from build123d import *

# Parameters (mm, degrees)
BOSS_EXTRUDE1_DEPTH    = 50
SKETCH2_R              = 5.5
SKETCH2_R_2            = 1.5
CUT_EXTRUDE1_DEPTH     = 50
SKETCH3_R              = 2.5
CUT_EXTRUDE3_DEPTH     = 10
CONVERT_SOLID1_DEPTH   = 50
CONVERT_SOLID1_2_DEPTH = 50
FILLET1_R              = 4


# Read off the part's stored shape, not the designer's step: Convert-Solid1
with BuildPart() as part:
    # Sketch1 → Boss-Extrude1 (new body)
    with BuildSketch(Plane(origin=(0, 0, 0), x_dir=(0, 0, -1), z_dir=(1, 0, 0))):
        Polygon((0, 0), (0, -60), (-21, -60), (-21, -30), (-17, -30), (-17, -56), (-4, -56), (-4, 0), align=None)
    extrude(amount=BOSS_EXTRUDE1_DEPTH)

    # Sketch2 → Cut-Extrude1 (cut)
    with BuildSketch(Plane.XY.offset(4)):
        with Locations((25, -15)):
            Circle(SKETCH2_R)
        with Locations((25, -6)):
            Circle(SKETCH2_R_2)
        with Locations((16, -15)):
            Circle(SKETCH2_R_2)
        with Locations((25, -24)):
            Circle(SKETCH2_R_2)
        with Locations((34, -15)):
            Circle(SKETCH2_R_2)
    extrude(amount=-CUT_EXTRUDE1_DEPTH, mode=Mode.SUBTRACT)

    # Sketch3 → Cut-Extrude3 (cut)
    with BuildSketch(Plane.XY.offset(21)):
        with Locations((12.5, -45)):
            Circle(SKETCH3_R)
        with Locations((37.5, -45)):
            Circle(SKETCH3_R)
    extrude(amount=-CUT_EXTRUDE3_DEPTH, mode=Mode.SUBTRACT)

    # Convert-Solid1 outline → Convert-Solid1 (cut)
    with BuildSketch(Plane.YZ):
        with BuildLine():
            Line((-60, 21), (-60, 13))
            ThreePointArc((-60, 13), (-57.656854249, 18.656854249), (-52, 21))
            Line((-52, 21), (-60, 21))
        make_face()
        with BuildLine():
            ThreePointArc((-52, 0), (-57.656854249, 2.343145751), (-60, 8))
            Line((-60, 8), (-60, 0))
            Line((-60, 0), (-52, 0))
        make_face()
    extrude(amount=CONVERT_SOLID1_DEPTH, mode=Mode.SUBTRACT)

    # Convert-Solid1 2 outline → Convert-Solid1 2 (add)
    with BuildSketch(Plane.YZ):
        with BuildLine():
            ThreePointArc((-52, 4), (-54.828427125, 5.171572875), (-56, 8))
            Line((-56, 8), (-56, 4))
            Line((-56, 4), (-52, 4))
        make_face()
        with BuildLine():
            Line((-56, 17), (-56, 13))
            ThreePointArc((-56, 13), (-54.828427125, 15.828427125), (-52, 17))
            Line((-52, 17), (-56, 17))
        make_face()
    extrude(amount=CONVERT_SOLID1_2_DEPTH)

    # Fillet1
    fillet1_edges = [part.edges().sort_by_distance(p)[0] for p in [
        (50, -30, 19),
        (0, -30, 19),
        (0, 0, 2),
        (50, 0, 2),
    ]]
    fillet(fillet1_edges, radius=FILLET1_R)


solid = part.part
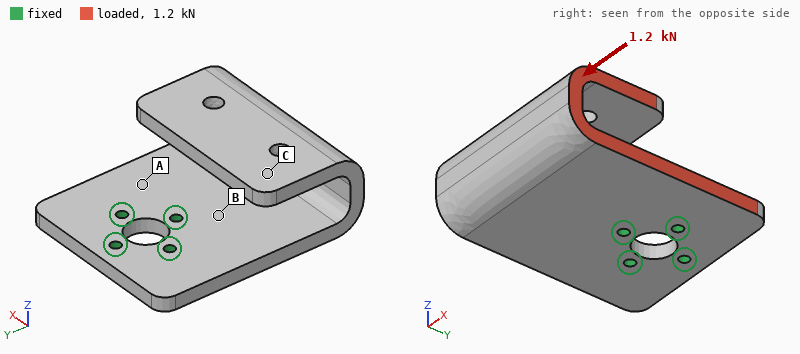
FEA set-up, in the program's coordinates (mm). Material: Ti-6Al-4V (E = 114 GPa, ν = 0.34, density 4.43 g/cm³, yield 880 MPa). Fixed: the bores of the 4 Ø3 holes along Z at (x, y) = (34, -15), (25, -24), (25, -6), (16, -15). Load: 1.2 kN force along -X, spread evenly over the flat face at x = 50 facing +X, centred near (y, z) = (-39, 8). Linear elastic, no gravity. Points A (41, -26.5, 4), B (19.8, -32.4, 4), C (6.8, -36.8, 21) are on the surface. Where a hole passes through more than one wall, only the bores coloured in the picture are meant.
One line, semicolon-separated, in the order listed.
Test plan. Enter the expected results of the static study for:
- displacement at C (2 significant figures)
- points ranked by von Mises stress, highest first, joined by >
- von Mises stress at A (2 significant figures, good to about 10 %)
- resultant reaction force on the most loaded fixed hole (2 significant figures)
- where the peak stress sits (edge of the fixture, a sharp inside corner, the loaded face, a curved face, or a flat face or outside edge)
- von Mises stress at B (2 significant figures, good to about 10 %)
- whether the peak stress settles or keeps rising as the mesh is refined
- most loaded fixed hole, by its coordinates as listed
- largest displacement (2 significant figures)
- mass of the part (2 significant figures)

0.15 mm; B > A > C; 30 MPa; 1.2 kN; edge of the fixture; 51 MPa; keeps rising; (25, -24); 0.17 mm; 84 g
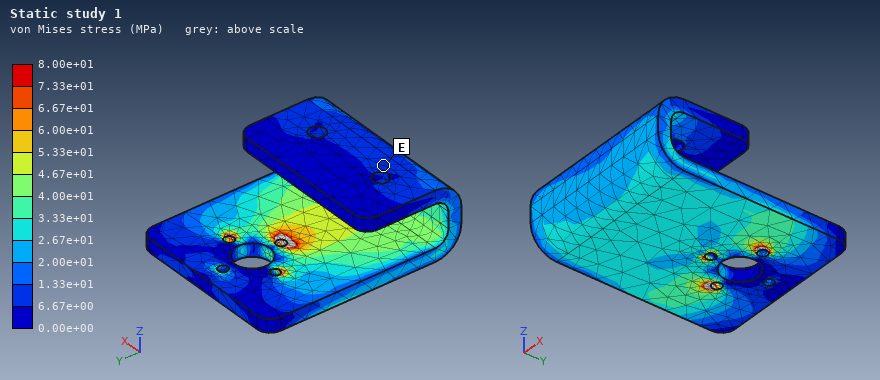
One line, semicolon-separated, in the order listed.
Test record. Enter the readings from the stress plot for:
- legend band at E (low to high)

6.67e+00 to 1.33e+01 MPa
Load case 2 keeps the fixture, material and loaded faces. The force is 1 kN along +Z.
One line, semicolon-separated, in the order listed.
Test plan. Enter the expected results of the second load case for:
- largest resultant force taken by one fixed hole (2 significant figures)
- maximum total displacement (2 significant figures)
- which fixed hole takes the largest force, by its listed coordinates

1.2 kN; 0.55 mm; (25, -24)
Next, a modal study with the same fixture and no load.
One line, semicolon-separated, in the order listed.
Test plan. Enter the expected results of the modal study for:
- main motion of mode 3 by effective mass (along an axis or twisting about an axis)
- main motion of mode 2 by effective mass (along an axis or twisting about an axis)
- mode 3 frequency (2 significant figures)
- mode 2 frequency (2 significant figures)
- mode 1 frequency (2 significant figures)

along Z; along X; 1800 Hz; 1400 Hz; 1100 Hz
